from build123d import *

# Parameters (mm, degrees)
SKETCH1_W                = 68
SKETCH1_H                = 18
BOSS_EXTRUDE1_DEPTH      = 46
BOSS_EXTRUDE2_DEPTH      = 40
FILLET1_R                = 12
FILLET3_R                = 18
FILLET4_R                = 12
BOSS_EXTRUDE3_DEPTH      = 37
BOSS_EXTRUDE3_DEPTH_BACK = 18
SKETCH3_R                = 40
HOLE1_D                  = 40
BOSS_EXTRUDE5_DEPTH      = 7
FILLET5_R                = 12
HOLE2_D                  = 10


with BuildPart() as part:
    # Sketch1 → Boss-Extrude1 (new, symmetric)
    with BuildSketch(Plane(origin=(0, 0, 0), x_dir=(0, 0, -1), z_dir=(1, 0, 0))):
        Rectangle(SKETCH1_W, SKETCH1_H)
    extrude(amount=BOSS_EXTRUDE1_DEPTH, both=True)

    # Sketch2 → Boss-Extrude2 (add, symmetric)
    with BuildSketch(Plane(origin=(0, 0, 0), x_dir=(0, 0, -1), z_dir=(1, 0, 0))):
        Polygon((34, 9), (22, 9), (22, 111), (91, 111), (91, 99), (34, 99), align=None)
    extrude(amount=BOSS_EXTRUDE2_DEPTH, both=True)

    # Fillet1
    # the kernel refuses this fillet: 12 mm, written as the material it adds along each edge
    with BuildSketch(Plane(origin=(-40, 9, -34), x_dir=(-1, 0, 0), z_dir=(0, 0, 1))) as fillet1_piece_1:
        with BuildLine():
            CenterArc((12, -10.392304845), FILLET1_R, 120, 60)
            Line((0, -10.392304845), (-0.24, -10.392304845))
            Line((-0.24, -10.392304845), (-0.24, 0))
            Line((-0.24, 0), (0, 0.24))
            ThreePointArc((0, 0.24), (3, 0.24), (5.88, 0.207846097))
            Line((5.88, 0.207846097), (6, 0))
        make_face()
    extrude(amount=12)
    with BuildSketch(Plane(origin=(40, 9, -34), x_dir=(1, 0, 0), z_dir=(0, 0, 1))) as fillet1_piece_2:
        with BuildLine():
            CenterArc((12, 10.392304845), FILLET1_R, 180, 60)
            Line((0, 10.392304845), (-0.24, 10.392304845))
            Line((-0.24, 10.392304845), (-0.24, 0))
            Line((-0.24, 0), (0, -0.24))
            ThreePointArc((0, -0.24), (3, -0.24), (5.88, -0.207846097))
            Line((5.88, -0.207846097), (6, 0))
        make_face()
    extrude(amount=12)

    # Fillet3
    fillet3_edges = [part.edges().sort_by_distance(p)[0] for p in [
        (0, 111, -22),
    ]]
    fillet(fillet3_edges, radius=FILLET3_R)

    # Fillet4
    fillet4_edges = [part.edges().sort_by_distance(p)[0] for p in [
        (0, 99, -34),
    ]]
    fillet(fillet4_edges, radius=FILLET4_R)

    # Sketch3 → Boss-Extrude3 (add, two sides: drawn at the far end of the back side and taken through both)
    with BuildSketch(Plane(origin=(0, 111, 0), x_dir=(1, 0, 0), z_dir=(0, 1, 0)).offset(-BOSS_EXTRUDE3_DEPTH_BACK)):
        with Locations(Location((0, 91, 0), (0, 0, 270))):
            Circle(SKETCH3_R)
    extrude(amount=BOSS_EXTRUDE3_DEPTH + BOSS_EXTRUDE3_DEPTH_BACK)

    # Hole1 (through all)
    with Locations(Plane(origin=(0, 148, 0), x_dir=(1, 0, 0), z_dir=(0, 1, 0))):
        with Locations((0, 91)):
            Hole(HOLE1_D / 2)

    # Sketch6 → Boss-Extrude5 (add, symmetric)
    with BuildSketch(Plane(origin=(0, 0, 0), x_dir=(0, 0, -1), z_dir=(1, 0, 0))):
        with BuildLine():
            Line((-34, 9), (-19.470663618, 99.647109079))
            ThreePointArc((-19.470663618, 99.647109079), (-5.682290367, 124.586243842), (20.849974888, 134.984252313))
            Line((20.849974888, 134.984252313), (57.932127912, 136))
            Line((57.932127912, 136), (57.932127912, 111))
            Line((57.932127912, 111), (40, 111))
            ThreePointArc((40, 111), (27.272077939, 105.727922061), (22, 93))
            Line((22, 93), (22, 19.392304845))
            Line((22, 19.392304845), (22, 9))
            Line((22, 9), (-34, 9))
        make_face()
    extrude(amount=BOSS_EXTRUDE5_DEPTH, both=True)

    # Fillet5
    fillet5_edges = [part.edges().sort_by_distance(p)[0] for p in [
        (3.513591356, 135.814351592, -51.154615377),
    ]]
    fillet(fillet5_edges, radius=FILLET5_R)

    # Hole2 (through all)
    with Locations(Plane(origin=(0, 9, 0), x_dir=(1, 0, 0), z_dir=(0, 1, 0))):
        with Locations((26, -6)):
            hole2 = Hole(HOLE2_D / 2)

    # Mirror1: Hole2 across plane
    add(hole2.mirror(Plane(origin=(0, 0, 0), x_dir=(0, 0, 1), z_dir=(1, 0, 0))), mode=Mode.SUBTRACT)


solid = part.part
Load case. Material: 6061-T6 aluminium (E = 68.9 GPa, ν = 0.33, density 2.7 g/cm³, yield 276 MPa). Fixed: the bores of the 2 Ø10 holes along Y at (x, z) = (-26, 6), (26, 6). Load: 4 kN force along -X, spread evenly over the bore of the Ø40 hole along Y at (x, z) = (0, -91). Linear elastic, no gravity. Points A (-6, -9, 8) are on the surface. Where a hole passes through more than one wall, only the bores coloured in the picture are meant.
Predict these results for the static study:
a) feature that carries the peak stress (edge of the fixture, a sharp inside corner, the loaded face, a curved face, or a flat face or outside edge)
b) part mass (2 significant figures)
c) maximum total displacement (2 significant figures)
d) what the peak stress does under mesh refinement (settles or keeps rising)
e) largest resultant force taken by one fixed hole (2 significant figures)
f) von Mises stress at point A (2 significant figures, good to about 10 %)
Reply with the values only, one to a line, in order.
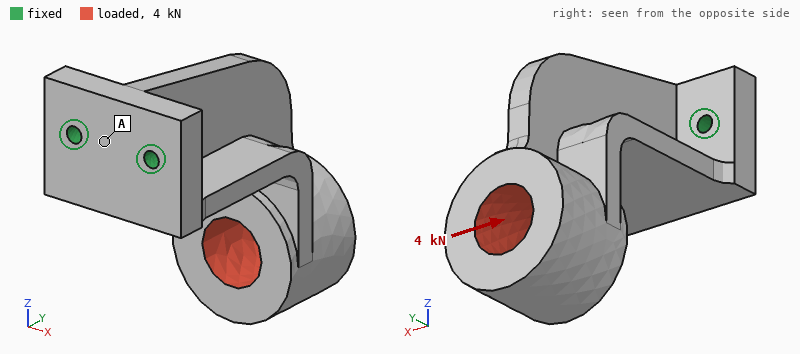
edge of the fixture
1.4 kg
1.1 mm
keeps rising
10 kN
14 MPa
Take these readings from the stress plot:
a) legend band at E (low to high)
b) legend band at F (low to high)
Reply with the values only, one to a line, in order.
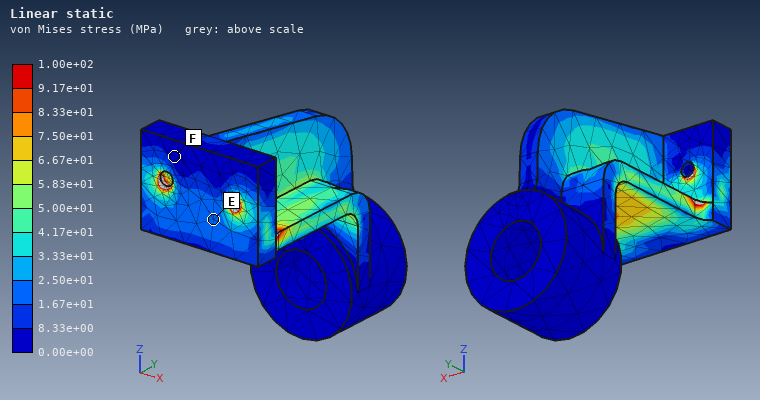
1.67e+01 to 2.50e+01 MPa
0.00e+00 to 8.33e+00 MPa
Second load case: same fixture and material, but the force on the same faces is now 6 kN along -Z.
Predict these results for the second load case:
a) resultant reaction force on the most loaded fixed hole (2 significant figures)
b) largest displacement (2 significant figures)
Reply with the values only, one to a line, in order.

3.0 kN
0.77 mm
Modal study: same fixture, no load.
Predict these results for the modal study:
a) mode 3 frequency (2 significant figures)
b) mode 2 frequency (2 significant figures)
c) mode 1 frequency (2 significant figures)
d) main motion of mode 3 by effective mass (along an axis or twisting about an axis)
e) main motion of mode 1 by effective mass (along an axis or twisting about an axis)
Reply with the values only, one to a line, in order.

1100 Hz
520 Hz
440 Hz
along X
along X
